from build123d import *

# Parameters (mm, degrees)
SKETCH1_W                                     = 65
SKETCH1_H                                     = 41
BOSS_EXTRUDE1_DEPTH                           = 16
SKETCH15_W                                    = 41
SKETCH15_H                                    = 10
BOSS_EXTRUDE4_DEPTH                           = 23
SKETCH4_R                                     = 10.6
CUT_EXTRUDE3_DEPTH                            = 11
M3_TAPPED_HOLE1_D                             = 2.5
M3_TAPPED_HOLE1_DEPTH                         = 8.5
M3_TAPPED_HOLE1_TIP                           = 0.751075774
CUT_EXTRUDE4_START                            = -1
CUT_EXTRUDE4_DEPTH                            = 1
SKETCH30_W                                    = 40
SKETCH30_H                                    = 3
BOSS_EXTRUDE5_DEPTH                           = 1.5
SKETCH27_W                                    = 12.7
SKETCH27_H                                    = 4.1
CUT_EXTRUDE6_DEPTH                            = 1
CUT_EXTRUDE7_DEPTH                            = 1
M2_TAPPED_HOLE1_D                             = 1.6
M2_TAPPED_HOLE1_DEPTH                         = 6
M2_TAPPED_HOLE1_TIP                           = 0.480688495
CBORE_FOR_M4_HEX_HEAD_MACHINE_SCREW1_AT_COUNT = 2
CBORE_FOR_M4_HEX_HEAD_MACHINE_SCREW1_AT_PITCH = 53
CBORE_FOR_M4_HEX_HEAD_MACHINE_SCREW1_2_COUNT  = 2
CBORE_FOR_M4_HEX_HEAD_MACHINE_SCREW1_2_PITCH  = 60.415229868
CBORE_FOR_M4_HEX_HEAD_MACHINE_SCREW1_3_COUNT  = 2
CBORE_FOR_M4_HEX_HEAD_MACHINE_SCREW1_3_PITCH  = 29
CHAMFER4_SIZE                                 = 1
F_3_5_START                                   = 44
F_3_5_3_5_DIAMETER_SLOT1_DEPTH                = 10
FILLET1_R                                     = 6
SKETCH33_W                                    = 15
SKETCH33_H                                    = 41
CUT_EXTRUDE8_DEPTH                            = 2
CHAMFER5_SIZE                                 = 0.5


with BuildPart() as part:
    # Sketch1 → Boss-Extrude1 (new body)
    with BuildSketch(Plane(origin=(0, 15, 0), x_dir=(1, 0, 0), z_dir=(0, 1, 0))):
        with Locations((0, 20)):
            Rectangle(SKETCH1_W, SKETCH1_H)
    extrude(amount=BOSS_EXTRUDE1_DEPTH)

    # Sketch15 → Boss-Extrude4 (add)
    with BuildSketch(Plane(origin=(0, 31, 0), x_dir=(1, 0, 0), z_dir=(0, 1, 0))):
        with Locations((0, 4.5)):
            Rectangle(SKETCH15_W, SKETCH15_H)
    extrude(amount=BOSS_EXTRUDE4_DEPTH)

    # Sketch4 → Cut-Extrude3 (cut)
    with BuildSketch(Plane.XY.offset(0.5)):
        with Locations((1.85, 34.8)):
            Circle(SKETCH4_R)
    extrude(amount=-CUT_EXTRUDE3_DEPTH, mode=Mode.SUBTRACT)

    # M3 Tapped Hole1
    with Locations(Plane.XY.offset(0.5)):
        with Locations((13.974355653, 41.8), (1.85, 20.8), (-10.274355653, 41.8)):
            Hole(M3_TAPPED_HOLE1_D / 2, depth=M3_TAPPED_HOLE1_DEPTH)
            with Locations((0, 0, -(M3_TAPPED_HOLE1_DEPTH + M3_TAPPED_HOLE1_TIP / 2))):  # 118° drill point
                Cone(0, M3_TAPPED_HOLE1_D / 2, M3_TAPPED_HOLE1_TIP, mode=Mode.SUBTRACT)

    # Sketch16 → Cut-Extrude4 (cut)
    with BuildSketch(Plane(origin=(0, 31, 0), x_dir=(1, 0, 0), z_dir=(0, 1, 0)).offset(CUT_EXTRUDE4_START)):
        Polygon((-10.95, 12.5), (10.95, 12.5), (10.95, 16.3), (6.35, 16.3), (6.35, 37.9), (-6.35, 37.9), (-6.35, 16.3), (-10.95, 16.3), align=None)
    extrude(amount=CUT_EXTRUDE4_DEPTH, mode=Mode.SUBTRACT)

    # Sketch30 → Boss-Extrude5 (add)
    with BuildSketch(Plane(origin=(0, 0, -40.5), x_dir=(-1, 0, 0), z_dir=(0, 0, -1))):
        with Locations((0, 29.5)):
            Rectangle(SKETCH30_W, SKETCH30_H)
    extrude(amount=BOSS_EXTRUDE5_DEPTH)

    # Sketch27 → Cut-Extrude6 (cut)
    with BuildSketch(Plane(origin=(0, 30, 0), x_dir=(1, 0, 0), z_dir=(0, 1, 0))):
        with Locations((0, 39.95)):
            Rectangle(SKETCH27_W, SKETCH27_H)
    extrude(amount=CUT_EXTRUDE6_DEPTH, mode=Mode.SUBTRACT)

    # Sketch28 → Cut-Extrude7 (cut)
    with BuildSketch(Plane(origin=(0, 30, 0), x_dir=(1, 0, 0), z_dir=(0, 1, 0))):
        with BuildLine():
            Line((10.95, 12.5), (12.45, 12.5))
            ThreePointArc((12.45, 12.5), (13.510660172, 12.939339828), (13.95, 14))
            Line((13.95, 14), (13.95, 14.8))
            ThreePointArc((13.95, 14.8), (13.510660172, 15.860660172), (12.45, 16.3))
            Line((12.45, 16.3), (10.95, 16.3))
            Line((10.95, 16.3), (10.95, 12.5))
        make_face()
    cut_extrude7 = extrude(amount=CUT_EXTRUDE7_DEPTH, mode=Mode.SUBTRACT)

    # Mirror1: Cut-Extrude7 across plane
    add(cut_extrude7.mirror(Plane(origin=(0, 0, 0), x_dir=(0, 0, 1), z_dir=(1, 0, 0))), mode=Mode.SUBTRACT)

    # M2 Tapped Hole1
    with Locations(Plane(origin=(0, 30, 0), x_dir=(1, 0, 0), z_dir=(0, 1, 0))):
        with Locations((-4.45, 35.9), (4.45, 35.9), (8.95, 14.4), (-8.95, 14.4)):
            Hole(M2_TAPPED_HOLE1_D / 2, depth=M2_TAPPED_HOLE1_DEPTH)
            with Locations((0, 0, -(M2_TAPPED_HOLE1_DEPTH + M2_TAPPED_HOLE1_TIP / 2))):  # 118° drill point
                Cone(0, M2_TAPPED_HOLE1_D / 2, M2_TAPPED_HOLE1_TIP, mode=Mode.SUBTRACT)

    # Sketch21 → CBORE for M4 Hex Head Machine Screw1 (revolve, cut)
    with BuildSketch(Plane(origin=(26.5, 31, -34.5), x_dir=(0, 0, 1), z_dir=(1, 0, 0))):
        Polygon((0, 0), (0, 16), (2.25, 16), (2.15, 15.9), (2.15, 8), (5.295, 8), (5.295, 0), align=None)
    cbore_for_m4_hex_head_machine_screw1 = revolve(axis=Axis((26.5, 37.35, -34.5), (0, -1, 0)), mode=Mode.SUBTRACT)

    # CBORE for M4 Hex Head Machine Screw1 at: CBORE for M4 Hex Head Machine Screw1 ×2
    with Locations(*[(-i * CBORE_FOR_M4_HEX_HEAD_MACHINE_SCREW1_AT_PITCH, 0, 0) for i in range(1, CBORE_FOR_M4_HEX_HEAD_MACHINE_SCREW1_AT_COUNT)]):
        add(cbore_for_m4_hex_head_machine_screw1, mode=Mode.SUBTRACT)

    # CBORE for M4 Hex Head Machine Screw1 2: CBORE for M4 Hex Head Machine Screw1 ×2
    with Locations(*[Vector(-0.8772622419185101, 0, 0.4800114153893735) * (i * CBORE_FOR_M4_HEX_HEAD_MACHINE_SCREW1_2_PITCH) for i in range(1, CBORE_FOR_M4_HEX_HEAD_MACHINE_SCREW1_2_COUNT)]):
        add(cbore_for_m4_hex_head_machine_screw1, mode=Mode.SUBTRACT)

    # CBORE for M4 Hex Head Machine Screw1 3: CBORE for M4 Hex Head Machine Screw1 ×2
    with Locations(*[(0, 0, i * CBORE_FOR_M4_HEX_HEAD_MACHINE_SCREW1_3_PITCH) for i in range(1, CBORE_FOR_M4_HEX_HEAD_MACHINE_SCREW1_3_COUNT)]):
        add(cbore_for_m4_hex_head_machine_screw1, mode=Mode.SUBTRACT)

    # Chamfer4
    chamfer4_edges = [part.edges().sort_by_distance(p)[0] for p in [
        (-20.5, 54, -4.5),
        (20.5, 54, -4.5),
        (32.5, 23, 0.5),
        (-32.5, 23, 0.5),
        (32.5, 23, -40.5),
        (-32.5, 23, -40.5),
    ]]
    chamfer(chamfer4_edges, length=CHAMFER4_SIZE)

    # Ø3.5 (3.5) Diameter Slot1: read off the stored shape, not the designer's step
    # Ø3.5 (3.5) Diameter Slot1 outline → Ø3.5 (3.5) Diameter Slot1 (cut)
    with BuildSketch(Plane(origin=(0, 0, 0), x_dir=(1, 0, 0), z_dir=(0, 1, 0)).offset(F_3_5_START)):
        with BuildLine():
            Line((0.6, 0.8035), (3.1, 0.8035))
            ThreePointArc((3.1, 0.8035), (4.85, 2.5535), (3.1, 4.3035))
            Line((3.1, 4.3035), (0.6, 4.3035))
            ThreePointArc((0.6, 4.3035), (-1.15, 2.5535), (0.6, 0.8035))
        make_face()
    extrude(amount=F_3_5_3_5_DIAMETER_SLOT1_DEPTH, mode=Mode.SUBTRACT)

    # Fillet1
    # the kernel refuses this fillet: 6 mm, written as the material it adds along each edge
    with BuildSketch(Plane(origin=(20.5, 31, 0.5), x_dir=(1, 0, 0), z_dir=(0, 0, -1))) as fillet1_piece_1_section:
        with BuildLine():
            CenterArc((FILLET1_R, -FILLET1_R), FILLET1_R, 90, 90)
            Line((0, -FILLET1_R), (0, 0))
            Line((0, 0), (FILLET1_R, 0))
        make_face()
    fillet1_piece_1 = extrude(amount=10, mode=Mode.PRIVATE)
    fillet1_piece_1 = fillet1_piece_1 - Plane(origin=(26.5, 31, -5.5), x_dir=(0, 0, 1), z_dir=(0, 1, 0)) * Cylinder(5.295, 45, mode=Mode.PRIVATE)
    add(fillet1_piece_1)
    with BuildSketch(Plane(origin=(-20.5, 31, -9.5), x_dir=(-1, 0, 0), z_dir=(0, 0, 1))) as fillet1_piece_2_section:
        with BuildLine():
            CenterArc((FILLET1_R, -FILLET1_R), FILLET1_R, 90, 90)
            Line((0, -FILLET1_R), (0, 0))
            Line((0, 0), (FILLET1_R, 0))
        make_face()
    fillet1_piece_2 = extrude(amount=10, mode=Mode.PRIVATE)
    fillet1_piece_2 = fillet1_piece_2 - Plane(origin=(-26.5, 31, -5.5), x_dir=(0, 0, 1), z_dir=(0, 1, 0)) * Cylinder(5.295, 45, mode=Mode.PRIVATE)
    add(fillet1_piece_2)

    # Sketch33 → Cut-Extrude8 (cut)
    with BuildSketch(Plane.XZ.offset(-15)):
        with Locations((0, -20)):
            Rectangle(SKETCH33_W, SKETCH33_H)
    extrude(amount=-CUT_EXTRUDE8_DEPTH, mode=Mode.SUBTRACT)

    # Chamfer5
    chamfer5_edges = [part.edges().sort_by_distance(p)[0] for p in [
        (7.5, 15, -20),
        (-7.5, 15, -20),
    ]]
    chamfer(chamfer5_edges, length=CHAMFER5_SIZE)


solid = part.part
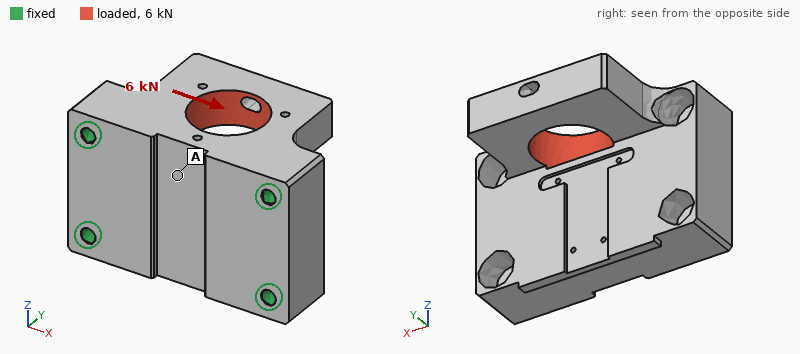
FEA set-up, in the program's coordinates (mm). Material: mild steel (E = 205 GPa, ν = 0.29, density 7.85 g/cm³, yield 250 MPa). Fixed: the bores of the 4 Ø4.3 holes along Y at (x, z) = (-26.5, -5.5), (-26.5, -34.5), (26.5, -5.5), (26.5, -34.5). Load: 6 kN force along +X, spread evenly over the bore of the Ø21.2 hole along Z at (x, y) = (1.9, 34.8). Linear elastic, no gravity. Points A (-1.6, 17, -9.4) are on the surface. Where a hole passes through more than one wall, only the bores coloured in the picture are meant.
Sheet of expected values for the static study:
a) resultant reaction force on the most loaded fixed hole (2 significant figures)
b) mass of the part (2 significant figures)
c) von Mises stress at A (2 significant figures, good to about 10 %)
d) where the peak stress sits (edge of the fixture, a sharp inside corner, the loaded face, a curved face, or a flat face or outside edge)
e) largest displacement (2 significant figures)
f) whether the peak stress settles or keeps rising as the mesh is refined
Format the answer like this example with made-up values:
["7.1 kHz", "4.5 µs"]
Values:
["2.6 kN", "340 g", "11 MPa", "a sharp inside corner", "10 µm", "keeps rising"]
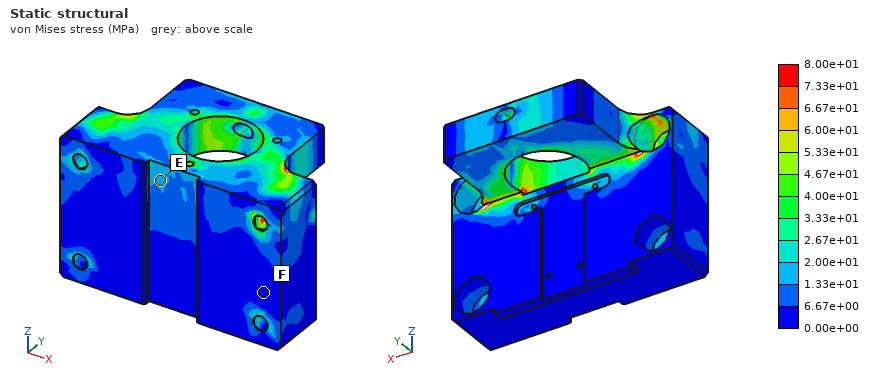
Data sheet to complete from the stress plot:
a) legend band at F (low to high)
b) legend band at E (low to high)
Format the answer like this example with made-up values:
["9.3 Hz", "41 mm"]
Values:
["0.00e+00 to 6.67e+00 MPa", "1.33e+01 to 2.00e+01 MPa"]
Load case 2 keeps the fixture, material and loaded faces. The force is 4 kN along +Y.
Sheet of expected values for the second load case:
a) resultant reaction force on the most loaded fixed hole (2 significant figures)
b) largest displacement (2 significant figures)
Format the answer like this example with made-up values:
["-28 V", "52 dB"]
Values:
["2.3 kN", "5.7 µm"]
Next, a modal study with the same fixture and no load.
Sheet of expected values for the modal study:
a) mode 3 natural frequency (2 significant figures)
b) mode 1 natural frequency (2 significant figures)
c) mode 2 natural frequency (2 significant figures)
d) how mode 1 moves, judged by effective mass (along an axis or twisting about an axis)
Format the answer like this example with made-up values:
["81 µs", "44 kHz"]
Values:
["13 kHz", "7200 Hz", "13 kHz", "along Z"]
